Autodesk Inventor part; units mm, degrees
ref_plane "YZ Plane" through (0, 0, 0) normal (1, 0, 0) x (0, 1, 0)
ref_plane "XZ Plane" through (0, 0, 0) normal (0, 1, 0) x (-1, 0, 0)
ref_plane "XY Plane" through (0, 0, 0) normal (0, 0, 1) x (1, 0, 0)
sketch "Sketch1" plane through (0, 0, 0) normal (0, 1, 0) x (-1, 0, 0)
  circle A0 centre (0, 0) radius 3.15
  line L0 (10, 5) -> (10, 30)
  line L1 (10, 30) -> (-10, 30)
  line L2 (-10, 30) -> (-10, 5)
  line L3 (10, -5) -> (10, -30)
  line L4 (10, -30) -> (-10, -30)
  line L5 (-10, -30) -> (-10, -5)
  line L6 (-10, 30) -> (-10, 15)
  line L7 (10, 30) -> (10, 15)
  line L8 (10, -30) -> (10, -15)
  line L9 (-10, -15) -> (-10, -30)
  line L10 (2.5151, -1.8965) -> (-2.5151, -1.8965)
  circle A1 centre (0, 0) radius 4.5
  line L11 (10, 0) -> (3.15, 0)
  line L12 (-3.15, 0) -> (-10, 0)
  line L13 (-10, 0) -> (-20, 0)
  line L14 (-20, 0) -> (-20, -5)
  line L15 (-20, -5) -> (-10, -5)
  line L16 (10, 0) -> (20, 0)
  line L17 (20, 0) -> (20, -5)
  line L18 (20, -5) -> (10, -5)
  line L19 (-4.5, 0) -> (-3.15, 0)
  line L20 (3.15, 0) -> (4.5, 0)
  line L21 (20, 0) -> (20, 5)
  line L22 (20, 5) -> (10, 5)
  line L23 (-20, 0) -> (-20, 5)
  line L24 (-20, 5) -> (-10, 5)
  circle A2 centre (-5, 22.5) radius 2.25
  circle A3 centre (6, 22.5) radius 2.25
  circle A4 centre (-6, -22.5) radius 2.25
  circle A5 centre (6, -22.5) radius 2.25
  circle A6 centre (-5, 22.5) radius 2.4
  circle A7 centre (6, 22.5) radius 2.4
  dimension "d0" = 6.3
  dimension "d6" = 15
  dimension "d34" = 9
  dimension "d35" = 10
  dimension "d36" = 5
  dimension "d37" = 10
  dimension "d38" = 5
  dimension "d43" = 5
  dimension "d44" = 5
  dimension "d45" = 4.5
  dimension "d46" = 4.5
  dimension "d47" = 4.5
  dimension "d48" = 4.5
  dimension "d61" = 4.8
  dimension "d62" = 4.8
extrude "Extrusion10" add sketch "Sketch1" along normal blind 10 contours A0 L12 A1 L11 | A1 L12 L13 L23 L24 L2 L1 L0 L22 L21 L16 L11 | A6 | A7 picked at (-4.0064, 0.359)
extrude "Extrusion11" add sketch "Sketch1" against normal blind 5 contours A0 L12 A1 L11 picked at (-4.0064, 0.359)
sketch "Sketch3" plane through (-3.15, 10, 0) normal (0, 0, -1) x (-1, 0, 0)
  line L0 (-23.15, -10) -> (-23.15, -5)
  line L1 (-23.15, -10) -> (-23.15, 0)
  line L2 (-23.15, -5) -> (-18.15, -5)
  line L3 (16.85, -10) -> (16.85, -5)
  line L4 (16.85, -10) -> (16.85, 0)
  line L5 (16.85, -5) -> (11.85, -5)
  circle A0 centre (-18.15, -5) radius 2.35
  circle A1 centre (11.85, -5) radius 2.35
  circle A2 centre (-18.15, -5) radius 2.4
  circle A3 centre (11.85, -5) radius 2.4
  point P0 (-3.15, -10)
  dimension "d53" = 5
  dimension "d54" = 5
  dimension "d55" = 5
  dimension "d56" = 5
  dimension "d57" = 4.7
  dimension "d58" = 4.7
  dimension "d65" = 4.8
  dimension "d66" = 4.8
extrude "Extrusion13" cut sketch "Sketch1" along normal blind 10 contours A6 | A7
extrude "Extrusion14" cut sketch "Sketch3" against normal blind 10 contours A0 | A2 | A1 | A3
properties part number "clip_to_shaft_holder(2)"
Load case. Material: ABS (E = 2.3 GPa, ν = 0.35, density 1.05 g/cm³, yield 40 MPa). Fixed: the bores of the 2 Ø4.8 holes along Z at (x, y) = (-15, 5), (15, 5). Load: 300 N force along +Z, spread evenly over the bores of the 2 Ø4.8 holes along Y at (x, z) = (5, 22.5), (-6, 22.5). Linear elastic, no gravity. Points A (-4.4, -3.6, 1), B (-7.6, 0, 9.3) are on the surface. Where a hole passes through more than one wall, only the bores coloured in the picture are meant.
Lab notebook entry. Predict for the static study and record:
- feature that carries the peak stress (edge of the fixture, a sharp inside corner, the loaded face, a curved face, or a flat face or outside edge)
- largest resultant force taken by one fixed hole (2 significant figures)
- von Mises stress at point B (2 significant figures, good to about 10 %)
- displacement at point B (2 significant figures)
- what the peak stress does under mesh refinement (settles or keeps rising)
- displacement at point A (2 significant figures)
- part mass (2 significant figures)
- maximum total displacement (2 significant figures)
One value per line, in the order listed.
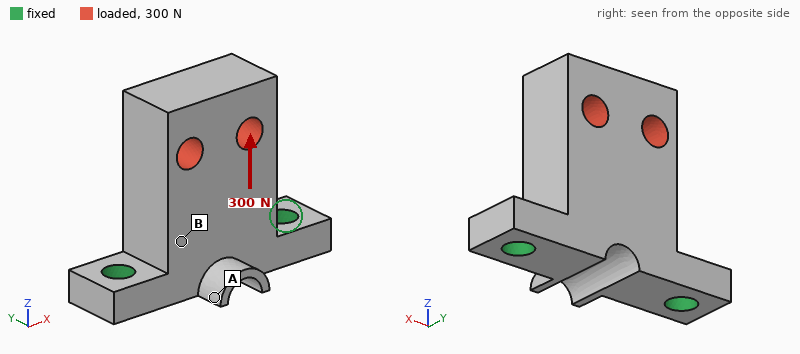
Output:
edge of the fixture
180 N
3.0 MPa
38 µm
keeps rising
41 µm
6.7 g
53 µm
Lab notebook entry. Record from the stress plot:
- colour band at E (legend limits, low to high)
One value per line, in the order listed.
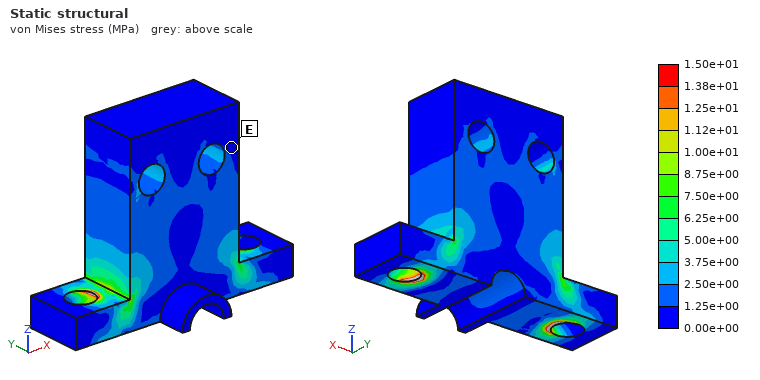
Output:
0.00e+00 to 1.25e+00 MPa
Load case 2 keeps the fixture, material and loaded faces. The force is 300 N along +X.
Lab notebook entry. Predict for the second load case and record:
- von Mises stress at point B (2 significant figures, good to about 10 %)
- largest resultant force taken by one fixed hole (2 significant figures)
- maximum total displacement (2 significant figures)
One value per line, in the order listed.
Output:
5.7 MPa
300 N
0.24 mm
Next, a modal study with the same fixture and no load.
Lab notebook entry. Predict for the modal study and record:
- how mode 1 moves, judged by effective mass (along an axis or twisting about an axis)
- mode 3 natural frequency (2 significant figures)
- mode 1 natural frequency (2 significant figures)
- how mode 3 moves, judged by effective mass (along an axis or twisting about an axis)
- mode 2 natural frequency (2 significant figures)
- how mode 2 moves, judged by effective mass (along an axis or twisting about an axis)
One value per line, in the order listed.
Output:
along Y
5700 Hz
1300 Hz
along Z
3600 Hz
along X
